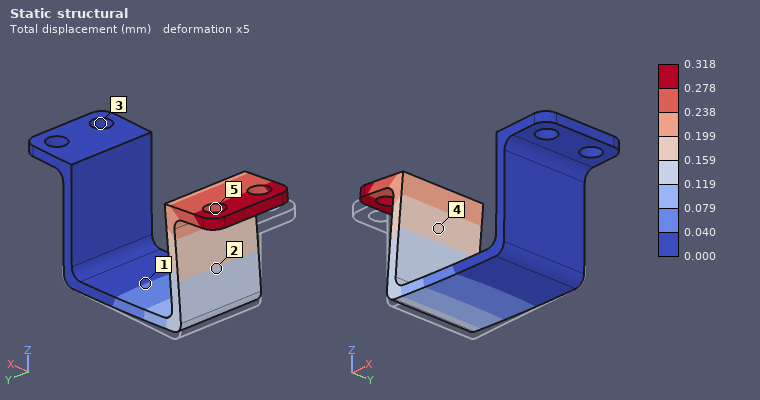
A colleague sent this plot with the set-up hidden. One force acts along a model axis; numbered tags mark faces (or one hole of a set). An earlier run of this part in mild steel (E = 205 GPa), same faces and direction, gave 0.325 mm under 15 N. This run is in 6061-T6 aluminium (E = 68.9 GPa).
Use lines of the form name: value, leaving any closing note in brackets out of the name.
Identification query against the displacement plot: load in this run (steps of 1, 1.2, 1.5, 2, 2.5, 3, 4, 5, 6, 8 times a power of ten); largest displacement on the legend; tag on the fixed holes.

load in this run: 5 N
largest displacement on the legend: 0.318 mm
tag on the fixed holes: 3
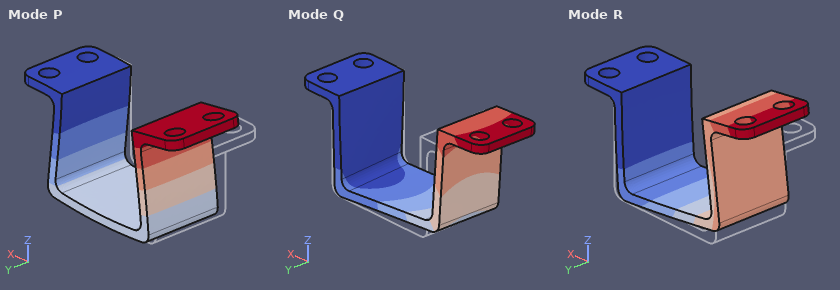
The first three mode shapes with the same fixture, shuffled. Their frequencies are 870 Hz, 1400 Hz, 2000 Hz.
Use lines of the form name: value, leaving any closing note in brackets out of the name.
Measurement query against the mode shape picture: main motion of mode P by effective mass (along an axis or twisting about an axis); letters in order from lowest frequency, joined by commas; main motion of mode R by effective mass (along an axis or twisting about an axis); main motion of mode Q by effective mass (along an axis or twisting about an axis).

main motion of mode P by effective mass: along X
letters in order from lowest frequency, joined by commas: R, Q, P
main motion of mode R by effective mass: along Z
main motion of mode Q by effective mass: along Y
